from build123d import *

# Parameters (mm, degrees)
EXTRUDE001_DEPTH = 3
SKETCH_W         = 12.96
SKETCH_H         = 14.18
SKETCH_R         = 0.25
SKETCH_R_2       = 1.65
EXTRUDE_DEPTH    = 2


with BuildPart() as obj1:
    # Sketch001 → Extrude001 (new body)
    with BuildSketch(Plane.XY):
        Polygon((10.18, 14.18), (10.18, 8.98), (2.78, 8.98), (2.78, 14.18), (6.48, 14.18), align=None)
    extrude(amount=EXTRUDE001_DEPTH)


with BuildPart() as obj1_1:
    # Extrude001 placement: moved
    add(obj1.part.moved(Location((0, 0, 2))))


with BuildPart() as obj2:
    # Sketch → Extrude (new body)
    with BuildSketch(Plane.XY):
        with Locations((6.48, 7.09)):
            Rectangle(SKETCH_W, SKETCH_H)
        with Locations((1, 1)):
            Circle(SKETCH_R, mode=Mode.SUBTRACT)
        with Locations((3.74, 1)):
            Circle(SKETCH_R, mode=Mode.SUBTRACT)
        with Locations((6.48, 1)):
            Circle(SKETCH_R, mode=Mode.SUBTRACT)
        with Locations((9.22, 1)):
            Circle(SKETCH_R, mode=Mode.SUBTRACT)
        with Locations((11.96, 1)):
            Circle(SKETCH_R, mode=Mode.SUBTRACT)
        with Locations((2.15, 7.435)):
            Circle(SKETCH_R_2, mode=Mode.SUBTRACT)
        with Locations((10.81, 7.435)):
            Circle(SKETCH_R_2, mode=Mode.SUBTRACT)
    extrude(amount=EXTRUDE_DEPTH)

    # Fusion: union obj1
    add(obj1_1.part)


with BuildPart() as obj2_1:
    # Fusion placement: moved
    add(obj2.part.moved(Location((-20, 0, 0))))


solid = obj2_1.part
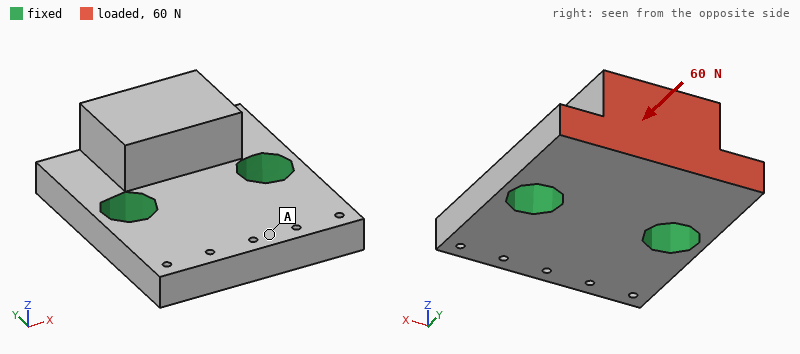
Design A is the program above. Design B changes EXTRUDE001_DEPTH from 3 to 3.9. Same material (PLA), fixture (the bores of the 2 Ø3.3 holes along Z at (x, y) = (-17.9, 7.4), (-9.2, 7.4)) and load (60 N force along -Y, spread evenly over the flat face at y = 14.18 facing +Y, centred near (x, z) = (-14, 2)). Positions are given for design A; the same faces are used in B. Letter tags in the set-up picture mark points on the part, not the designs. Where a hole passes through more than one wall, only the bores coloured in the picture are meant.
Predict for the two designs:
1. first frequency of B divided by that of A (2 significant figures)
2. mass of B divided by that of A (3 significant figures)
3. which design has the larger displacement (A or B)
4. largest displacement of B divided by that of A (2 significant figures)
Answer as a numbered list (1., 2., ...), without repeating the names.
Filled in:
1. 0.86
2. 1.08
3. B
4. 1.5
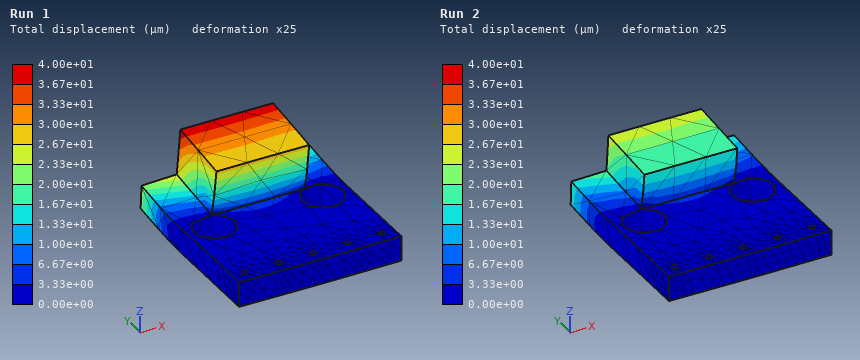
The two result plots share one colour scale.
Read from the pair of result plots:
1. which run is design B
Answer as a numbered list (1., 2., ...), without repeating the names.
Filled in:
1. Run 1
